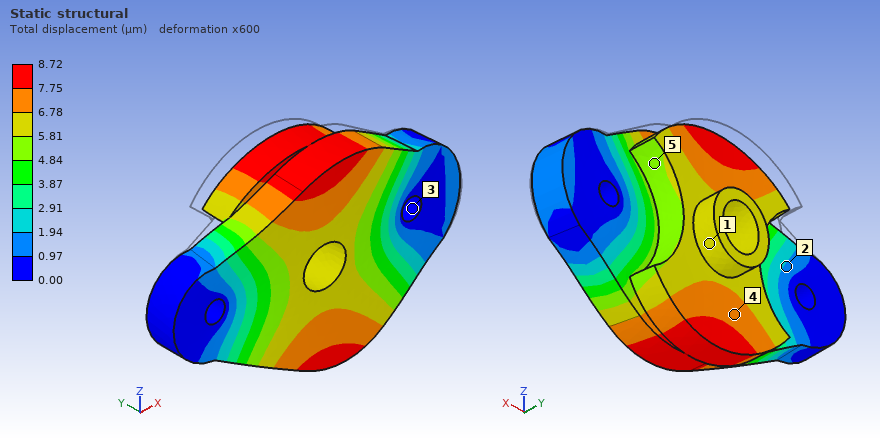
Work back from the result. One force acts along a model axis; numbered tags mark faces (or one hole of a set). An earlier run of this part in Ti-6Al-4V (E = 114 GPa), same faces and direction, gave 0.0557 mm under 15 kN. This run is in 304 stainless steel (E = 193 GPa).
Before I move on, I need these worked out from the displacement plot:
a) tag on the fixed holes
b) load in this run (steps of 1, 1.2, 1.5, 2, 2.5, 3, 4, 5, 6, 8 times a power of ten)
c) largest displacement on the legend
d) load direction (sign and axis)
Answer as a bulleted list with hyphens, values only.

- 3
- 4 kN
- 8.72 µm
- -Y
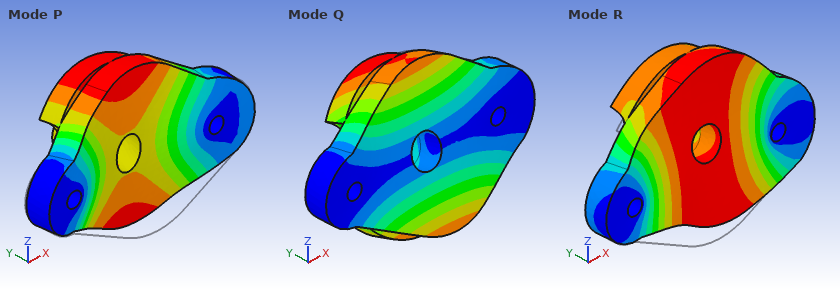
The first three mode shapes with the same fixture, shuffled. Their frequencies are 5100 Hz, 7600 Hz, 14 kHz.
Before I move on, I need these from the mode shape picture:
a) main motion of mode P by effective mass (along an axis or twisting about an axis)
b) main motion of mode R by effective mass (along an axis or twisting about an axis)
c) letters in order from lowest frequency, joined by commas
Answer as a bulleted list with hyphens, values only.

- along Y
- along Z
- Q, P, R
